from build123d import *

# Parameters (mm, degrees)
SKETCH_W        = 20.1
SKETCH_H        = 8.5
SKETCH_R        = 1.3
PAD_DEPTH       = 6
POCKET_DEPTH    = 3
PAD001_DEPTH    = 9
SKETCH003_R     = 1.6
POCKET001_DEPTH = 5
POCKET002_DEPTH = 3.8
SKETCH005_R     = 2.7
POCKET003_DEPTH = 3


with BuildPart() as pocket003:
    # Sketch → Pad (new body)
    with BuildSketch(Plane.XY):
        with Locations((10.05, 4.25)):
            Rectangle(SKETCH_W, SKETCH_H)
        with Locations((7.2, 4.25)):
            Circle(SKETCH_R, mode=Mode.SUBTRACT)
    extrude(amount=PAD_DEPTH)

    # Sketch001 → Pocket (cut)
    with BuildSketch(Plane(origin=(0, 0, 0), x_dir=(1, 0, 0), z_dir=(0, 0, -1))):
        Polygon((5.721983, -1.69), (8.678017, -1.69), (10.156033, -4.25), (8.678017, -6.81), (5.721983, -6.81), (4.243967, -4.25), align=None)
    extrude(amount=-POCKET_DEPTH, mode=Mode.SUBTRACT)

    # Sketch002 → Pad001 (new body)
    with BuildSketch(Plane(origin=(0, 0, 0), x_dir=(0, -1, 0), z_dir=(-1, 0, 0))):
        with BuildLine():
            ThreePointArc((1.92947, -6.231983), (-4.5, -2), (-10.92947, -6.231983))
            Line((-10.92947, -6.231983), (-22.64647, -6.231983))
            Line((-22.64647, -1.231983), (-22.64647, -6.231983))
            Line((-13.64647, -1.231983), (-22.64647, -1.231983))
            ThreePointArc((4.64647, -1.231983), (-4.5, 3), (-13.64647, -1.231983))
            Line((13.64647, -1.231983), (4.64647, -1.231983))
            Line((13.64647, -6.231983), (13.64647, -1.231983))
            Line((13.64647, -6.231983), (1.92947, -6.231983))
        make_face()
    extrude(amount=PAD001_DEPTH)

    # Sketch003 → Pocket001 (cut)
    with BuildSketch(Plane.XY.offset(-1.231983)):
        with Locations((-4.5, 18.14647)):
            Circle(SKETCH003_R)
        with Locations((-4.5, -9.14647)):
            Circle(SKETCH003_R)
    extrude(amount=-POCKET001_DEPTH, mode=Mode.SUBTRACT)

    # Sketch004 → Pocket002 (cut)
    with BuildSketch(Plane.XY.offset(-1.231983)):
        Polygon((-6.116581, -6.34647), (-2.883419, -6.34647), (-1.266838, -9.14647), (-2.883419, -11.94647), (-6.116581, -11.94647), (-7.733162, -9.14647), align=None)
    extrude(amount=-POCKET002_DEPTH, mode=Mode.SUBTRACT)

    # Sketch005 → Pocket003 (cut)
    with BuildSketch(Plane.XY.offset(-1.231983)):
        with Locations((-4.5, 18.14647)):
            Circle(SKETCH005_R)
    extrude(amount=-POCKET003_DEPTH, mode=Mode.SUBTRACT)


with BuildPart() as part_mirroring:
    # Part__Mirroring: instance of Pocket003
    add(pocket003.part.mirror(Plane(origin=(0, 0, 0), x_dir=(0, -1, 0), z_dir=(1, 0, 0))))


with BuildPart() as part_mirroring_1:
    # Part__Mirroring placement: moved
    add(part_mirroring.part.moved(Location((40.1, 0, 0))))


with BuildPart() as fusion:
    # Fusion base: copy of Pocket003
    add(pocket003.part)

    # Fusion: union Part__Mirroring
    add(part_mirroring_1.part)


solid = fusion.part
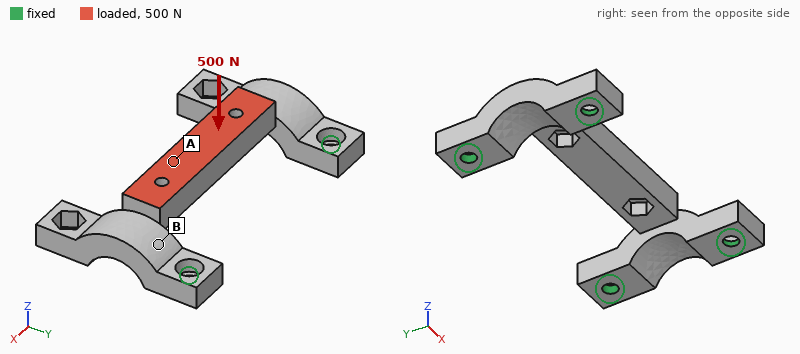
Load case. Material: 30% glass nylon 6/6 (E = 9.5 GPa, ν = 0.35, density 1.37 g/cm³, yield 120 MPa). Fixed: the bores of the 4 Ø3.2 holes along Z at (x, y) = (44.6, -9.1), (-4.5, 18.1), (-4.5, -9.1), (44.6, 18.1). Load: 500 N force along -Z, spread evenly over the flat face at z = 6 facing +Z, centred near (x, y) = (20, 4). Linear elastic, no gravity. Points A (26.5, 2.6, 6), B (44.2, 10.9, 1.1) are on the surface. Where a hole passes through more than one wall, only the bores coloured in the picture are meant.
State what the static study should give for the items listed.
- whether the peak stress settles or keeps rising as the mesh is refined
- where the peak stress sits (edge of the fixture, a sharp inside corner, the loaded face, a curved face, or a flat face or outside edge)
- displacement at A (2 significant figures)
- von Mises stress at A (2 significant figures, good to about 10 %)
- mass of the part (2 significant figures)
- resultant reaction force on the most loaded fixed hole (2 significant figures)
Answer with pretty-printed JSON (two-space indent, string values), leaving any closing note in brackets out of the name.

{
  "whether the peak stress settles or keeps rising as the mesh is refined": "keeps rising",
  "where the peak stress sits": "edge of the fixture",
  "displacement at A": "0.21 mm",
  "von Mises stress at A": "30 MPa",
  "mass of the part": "6.9 g",
  "resultant reaction force on the most loaded fixed hole": "240 N"
}
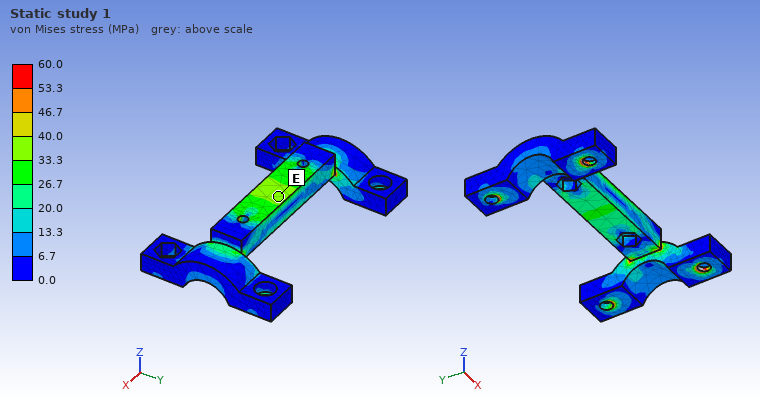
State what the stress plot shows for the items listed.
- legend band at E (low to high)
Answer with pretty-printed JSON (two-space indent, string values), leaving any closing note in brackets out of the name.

{
  "legend band at E": "33.3 to 40.0 MPa"
}
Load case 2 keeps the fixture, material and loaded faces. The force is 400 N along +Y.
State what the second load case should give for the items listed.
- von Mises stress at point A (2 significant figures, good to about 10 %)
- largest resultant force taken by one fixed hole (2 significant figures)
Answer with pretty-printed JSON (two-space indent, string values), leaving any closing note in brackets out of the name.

{
  "von Mises stress at point A": "8.5 MPa",
  "largest resultant force taken by one fixed hole": "160 N"
}
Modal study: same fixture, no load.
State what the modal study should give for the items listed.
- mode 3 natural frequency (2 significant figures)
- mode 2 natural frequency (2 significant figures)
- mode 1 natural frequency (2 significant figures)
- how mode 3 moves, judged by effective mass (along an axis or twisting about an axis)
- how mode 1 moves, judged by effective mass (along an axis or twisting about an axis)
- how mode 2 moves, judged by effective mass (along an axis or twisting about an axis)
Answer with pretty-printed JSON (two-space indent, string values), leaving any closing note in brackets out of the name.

{
  "mode 3 natural frequency": "6600 Hz",
  "mode 2 natural frequency": "5200 Hz",
  "mode 1 natural frequency": "5000 Hz",
  "how mode 3 moves, judged by effective mass": "along Y",
  "how mode 1 moves, judged by effective mass": "along Z",
  "how mode 2 moves, judged by effective mass": "along X"
}
